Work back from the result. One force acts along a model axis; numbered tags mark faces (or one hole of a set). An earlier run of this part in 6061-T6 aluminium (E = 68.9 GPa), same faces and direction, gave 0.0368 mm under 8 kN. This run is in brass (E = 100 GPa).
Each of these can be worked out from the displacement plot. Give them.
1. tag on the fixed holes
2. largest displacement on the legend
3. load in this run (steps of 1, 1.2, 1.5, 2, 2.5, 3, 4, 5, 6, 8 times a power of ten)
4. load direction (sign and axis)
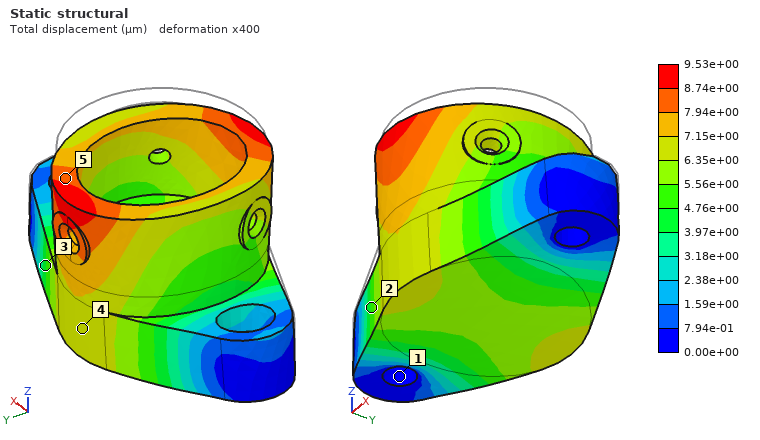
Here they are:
1
9.53e+00 µm
3 kN
-Z
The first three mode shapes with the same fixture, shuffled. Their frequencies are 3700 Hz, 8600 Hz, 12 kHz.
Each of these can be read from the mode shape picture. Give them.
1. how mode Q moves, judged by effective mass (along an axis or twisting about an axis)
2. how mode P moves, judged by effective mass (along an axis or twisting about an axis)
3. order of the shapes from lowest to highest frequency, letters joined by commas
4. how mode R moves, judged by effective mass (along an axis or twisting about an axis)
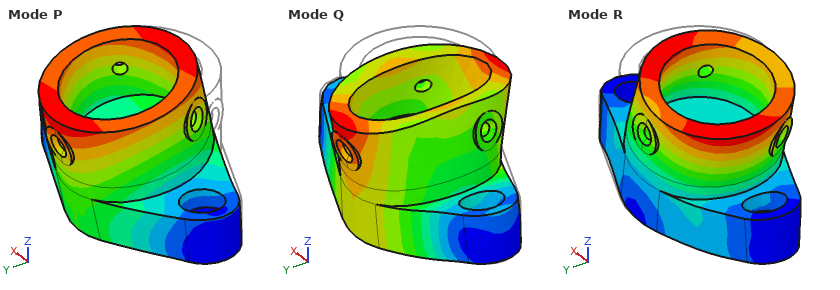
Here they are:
along Z
along Y
P, Q, R
along X
